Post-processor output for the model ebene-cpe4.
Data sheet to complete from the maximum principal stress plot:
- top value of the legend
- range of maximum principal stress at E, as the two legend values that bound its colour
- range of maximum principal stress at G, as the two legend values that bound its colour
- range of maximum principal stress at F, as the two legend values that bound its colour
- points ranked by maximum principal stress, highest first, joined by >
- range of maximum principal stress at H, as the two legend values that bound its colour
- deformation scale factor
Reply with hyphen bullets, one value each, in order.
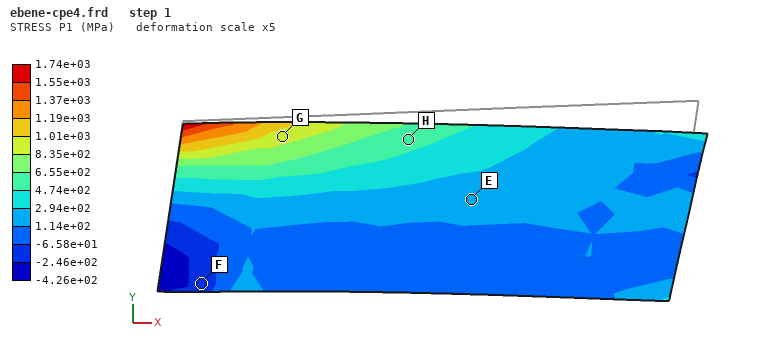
- 1.74e+03 MPa
- 1.14e+02 to 2.94e+02 MPa
- 8.35e+02 to 1.01e+03 MPa
- -2.46e+02 to -6.58e+01 MPa
- G > H > E > F
- 4.74e+02 to 6.55e+02 MPa
- 5
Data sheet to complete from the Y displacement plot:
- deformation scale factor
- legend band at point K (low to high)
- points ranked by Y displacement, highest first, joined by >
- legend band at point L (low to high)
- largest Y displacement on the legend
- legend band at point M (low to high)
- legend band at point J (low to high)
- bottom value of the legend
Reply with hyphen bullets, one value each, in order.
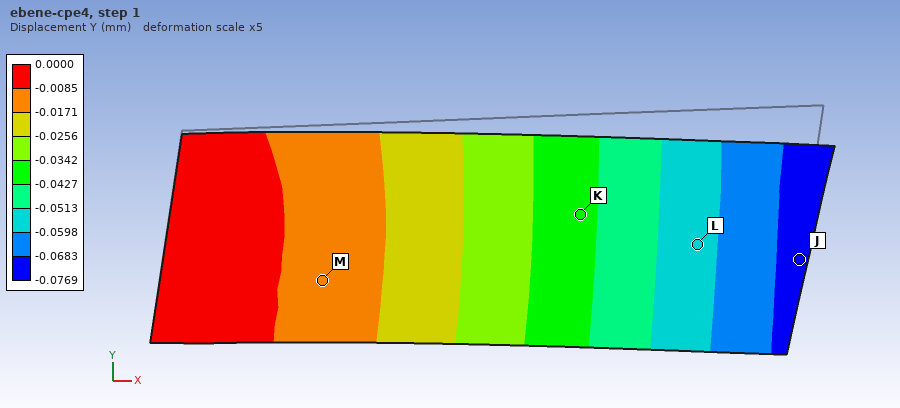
- 5
- -0.0427 to -0.0342 mm
- M > K > L > J
- -0.0598 to -0.0513 mm
- 0.0000 mm
- -0.0171 to -0.0085 mm
- -0.0769 to -0.0683 mm
- -0.0769 mm
